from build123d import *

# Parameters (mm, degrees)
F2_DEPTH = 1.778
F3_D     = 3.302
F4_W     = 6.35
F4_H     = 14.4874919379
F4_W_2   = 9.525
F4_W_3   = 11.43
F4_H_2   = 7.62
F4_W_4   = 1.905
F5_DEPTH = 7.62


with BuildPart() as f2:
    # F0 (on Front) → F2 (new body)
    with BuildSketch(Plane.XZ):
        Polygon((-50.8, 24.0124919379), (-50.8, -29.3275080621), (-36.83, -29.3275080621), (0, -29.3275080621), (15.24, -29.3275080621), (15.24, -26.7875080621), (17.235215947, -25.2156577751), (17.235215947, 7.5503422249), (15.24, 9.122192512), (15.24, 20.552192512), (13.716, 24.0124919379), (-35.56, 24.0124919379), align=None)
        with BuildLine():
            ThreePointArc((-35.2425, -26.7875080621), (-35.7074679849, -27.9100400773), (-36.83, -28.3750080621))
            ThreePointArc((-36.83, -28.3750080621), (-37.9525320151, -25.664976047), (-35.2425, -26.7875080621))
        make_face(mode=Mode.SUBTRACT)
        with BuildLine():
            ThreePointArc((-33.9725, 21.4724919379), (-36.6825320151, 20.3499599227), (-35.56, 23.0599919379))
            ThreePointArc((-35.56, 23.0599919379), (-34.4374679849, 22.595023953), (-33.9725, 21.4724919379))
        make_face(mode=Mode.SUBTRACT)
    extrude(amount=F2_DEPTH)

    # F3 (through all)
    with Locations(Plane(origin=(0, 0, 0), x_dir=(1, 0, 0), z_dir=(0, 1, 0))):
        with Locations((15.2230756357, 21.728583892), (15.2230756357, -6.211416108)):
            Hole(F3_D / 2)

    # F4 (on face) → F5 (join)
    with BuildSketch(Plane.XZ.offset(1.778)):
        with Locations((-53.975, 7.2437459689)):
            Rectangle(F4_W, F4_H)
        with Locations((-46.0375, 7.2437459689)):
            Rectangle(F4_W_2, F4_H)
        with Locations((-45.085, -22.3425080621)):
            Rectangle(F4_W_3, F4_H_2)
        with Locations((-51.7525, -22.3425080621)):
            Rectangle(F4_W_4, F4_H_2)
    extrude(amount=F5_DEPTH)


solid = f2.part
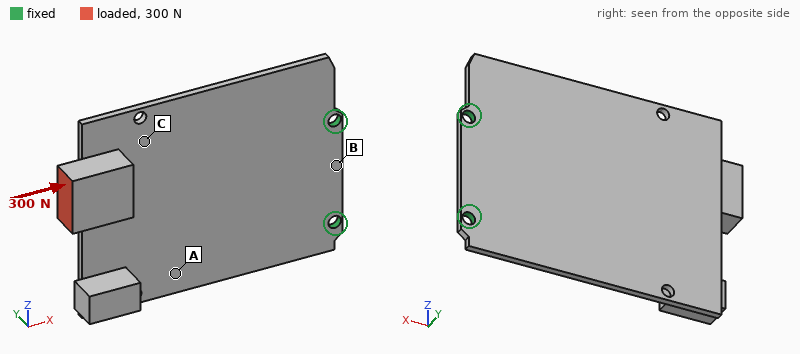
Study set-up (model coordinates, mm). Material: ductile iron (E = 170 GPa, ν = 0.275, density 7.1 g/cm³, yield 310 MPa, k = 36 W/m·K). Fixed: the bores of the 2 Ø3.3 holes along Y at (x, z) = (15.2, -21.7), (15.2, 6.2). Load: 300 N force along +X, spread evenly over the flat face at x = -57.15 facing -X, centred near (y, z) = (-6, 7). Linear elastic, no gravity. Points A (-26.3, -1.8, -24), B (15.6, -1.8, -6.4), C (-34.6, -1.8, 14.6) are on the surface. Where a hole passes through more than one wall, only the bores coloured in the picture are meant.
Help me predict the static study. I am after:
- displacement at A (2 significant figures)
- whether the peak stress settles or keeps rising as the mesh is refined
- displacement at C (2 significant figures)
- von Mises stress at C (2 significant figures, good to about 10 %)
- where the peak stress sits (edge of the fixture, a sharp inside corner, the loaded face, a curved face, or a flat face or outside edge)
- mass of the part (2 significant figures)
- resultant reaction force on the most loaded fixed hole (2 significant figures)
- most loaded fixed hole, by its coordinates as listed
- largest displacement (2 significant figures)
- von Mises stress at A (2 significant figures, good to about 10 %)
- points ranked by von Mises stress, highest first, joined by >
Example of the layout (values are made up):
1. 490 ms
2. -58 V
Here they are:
1. 0.31 mm
2. keeps rising
3. 0.47 mm
4. 67 MPa
5. edge of the fixture
6. 63 g
7. 310 N
8. (15.2, 6.2)
9. 0.96 mm
10. 43 MPa
11. C > A > B
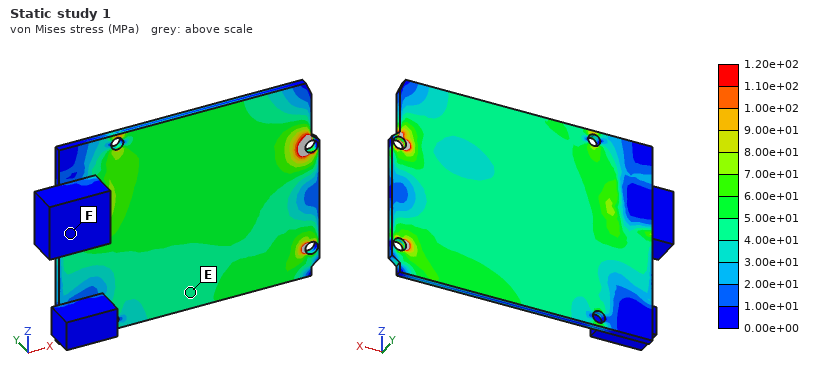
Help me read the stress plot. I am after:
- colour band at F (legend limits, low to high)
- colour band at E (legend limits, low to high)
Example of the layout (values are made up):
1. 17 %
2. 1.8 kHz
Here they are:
1. 0.00e+00 to 1.00e+01 MPa
2. 4.00e+01 to 5.00e+01 MPa
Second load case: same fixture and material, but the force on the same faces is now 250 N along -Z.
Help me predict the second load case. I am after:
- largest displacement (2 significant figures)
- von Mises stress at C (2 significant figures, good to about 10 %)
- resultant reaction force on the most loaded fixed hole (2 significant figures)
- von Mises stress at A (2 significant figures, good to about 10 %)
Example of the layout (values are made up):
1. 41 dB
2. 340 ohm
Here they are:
1. 0.26 mm
2. 38 MPa
3. 640 N
4. 28 MPa
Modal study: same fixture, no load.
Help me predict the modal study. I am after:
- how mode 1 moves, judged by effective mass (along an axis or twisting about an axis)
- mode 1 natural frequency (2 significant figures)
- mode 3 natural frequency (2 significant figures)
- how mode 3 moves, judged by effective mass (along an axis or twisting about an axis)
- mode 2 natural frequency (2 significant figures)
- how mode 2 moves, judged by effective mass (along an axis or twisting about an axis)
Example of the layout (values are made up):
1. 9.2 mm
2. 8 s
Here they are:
1. along Y
2. 190 Hz
3. 1400 Hz
4. along Y
5. 660 Hz
6. twisting about X
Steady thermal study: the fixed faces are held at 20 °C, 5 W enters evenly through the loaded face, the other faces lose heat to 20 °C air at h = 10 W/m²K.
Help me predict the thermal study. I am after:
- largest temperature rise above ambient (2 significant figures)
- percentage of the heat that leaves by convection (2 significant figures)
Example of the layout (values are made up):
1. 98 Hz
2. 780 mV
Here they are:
1. 82 K
2. 55 %
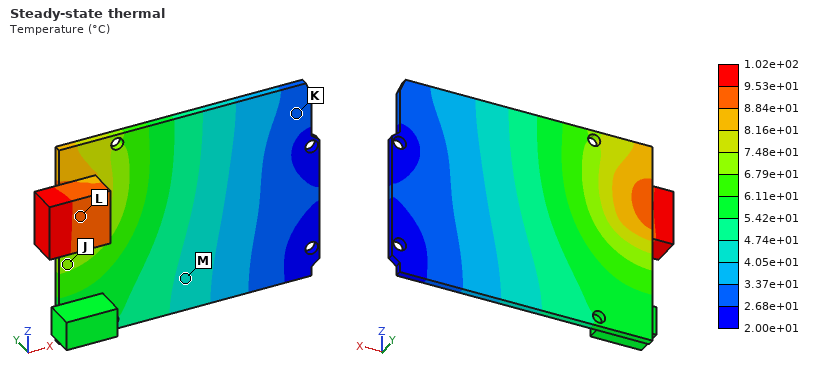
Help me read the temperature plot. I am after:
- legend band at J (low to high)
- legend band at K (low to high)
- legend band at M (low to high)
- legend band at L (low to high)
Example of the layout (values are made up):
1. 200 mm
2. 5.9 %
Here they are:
1. 6.79e+01 to 7.48e+01 °C
2. 2.68e+01 to 3.37e+01 °C
3. 4.05e+01 to 4.74e+01 °C
4. 8.84e+01 to 9.53e+01 °C
